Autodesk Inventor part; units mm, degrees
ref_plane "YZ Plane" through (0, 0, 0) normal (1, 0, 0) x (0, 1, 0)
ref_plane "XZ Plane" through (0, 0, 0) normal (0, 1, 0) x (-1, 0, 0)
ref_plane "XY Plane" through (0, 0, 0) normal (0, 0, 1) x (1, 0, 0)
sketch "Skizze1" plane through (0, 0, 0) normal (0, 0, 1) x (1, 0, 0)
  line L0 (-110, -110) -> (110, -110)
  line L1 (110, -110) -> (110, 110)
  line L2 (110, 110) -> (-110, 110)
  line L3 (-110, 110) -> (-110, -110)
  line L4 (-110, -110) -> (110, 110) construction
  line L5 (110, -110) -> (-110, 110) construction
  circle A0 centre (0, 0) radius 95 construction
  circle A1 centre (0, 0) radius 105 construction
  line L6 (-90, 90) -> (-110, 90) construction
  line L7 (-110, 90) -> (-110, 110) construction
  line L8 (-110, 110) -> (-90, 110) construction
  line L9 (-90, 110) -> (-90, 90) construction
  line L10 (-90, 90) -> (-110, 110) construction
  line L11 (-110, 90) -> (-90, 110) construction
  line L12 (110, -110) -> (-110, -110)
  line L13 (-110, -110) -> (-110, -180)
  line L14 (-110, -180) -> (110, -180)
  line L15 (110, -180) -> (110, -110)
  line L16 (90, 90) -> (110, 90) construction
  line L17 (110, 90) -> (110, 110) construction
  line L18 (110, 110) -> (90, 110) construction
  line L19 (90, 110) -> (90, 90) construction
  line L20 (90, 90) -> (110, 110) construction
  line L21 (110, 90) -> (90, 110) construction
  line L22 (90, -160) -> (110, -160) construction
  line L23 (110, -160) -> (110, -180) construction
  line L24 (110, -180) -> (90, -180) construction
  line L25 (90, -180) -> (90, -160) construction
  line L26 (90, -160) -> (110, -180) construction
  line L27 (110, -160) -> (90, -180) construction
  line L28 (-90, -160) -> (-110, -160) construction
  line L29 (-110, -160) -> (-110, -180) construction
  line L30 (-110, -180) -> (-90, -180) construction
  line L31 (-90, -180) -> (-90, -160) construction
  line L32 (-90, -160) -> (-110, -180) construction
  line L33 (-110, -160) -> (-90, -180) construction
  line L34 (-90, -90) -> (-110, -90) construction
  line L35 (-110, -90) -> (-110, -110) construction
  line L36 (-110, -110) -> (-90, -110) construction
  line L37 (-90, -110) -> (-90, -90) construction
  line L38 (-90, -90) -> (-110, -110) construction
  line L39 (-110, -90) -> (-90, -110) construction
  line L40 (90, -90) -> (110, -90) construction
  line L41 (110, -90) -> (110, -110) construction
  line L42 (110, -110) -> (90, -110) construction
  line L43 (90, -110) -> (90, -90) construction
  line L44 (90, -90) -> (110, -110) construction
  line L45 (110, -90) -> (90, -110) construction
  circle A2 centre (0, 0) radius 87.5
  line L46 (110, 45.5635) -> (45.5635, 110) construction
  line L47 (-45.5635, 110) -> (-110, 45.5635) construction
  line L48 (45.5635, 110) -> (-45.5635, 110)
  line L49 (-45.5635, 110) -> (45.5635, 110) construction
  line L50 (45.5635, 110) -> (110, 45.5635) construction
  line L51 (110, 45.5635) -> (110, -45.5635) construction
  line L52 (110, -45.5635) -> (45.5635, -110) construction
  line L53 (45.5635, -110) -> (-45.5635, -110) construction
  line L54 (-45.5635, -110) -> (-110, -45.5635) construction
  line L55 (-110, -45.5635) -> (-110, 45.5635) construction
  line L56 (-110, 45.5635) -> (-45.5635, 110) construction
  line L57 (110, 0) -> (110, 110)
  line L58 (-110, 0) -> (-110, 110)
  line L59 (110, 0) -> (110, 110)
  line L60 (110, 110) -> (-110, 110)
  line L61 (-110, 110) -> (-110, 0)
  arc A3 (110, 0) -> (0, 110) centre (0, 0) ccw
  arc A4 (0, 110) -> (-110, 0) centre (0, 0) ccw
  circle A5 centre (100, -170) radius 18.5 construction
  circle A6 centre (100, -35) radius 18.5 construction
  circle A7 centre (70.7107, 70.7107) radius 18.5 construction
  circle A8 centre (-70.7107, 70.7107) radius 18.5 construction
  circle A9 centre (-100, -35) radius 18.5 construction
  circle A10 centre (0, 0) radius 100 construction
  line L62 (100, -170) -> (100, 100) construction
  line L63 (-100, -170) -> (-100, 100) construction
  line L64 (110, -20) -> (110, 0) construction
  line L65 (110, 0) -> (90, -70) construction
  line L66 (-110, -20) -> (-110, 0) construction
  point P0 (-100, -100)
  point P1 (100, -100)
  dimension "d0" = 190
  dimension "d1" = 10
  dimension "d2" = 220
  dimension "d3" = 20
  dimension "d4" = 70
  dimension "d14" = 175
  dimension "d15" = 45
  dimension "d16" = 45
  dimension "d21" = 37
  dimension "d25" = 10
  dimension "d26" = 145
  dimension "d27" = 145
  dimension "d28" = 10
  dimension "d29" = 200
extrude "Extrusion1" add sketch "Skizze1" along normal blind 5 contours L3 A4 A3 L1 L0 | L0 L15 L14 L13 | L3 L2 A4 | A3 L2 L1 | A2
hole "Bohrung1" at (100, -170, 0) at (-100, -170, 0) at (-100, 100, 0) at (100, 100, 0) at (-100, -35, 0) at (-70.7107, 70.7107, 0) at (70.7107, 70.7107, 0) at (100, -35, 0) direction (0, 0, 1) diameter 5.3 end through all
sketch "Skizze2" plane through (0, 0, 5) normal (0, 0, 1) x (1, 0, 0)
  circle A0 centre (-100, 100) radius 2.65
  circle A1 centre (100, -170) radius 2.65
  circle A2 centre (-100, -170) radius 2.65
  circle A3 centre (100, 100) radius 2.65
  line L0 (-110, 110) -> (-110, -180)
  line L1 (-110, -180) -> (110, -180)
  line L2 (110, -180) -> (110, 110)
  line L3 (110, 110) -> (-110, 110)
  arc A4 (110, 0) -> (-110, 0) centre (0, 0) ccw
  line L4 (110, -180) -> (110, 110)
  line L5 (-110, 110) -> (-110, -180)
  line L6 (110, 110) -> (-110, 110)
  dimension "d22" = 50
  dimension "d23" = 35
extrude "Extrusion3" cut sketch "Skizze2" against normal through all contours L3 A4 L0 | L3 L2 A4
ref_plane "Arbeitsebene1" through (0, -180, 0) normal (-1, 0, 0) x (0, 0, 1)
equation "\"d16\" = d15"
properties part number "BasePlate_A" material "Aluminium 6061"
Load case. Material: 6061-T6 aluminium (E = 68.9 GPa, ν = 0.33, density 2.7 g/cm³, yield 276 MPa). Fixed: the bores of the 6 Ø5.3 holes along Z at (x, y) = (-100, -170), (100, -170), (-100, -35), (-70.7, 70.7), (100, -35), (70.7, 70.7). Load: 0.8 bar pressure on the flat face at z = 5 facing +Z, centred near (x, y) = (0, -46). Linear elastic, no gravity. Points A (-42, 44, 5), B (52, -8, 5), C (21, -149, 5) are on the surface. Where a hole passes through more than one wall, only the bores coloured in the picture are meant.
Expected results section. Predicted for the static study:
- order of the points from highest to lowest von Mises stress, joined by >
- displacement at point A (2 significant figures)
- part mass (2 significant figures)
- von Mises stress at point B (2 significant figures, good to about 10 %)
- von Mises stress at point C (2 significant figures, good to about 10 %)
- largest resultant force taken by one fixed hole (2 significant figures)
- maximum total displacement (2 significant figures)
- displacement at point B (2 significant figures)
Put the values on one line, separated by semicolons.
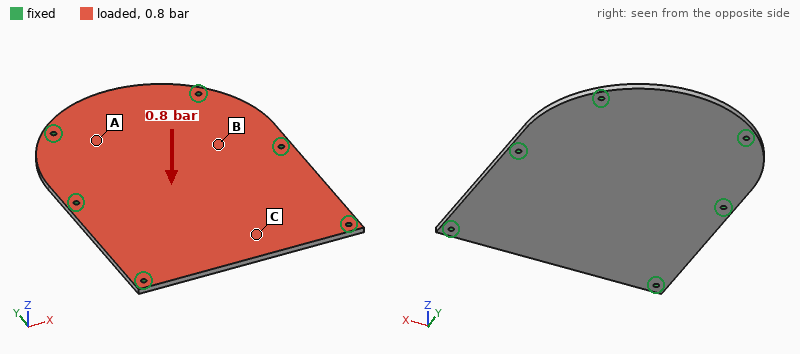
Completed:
C > B > A; 0.20 mm; 790 g; 18 MPa; 36 MPa; 1.0 kN; 0.79 mm; 0.32 mm
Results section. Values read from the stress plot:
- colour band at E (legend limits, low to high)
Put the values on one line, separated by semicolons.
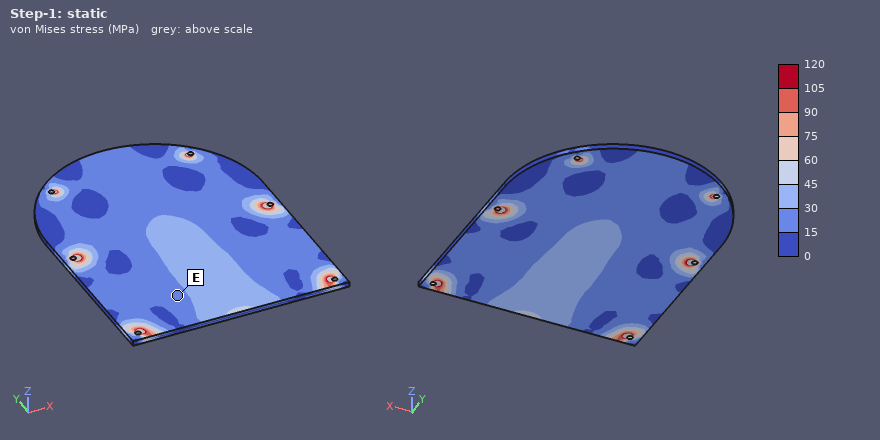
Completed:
15 to 30 MPa
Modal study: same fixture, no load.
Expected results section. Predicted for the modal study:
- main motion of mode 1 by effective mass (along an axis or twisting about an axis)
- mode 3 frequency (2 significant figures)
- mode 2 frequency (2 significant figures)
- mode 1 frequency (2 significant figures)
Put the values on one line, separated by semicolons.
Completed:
along Z; 1100 Hz; 820 Hz; 520 Hz
